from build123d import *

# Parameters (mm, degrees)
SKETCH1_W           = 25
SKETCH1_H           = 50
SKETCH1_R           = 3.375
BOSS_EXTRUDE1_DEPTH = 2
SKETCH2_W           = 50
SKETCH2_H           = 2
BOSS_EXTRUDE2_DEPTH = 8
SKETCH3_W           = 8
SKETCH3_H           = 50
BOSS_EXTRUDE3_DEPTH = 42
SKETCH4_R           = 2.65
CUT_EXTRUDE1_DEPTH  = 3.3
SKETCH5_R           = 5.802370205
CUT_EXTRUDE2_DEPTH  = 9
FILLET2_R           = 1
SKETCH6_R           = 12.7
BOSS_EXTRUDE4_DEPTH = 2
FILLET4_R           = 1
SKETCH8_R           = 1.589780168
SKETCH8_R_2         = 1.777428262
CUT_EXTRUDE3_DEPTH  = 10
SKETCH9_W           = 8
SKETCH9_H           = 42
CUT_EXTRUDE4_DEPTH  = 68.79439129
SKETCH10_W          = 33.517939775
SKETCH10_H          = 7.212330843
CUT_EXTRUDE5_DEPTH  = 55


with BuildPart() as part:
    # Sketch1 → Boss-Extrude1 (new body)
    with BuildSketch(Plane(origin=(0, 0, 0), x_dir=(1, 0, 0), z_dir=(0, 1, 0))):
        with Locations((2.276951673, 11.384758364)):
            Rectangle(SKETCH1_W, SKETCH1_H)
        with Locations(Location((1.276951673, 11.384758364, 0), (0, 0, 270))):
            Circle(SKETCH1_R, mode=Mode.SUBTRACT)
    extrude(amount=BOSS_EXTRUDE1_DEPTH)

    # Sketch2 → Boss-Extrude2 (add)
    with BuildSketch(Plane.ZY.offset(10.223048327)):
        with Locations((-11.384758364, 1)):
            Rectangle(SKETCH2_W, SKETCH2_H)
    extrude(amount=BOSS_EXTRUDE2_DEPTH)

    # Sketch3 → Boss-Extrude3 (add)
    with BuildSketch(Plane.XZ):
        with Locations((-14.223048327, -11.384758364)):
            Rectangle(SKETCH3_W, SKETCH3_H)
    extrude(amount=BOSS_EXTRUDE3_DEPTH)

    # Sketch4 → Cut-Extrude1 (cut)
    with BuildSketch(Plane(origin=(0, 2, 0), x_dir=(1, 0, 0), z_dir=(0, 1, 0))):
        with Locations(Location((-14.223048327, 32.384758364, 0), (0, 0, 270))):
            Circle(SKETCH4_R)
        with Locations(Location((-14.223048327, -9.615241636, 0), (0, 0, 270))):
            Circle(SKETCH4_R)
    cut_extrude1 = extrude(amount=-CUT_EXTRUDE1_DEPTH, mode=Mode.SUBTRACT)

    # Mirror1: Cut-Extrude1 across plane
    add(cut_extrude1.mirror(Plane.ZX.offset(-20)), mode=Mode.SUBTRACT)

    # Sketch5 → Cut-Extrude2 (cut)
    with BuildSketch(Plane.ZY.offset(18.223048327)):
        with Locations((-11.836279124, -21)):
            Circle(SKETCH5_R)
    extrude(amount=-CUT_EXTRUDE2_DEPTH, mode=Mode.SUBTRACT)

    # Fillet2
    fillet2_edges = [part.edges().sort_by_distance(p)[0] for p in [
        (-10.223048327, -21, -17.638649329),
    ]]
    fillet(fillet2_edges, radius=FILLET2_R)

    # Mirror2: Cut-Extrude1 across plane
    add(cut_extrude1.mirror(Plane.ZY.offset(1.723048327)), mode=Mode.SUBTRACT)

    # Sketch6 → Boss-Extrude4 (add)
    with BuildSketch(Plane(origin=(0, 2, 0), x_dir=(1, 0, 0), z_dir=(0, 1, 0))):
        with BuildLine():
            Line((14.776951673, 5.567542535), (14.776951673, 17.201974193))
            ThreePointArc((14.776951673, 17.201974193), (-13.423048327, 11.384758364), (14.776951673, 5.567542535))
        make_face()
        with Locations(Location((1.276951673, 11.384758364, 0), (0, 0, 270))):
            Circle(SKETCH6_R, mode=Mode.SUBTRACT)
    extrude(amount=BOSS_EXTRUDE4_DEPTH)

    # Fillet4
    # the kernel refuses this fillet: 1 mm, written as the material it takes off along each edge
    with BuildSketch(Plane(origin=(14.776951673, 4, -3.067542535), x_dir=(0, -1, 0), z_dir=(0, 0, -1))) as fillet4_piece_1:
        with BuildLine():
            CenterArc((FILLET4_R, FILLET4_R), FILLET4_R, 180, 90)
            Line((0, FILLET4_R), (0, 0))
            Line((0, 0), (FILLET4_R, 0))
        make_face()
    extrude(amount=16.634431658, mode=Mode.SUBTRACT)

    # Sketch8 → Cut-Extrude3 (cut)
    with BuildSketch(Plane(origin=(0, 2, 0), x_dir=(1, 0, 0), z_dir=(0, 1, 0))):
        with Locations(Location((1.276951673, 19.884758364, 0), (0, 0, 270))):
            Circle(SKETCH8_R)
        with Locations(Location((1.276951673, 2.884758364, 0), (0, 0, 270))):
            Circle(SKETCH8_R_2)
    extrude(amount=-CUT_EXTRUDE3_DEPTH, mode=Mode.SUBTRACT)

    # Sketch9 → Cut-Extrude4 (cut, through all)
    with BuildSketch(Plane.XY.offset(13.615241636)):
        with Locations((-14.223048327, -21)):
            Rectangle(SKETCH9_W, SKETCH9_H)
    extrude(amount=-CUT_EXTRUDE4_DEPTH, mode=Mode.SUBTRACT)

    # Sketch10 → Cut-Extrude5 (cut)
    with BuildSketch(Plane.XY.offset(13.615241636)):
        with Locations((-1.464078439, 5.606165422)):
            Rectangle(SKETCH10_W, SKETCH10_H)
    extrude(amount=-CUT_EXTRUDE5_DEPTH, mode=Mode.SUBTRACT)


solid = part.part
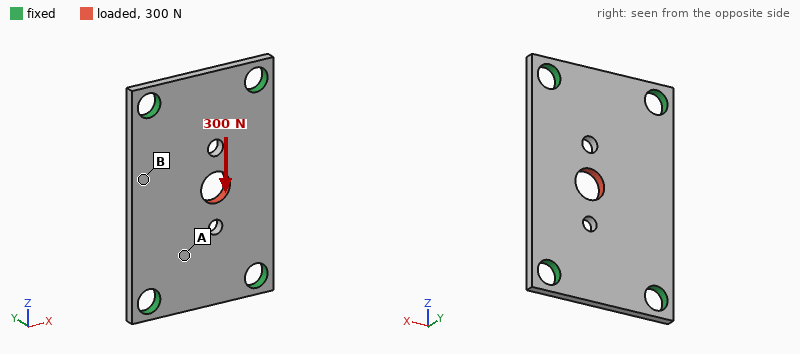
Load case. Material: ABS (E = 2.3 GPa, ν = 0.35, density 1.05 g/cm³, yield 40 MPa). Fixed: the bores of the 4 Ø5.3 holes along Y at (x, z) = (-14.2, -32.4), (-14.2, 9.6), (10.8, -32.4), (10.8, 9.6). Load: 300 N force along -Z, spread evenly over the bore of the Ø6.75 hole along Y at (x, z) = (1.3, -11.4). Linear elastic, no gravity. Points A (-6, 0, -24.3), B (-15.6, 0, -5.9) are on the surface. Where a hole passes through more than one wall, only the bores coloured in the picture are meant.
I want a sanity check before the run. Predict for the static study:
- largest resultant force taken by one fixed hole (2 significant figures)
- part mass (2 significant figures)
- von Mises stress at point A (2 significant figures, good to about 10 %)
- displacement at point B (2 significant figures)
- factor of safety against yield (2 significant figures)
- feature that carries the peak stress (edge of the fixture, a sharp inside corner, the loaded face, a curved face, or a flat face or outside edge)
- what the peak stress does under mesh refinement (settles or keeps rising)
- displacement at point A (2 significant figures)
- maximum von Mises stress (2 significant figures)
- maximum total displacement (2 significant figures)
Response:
90 N
3.2 g
3.2 MPa
8.8 µm
2.6
a curved face
settles
16 µm
15 MPa
46 µm
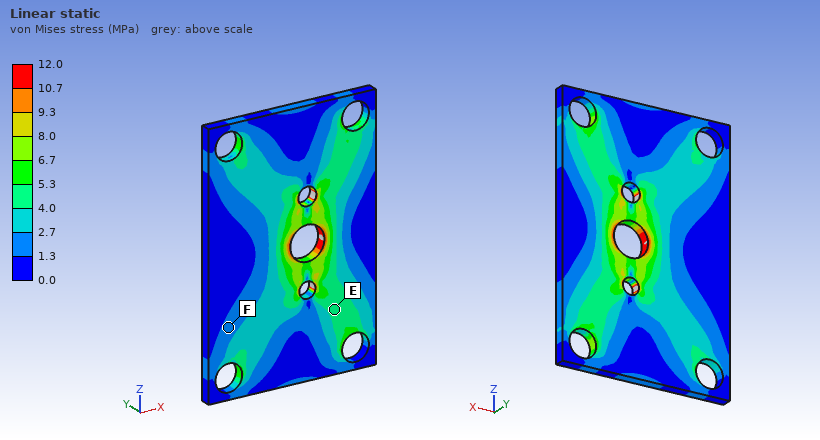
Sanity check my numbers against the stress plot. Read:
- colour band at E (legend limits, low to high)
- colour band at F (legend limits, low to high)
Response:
4.0 to 5.3 MPa
1.3 to 2.7 MPa
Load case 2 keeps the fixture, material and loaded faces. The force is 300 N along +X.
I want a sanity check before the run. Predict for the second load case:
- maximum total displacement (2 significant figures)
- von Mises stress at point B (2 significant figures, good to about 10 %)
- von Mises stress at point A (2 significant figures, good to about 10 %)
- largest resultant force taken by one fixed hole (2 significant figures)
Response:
83 µm
2.3 MPa
5.0 MPa
100 N
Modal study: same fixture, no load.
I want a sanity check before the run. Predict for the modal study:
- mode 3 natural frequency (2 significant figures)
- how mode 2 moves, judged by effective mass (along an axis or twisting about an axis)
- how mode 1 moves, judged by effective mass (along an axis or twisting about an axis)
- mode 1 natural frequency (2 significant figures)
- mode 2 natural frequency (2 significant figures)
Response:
4100 Hz
twisting about Z
along Y
1900 Hz
2600 Hz
